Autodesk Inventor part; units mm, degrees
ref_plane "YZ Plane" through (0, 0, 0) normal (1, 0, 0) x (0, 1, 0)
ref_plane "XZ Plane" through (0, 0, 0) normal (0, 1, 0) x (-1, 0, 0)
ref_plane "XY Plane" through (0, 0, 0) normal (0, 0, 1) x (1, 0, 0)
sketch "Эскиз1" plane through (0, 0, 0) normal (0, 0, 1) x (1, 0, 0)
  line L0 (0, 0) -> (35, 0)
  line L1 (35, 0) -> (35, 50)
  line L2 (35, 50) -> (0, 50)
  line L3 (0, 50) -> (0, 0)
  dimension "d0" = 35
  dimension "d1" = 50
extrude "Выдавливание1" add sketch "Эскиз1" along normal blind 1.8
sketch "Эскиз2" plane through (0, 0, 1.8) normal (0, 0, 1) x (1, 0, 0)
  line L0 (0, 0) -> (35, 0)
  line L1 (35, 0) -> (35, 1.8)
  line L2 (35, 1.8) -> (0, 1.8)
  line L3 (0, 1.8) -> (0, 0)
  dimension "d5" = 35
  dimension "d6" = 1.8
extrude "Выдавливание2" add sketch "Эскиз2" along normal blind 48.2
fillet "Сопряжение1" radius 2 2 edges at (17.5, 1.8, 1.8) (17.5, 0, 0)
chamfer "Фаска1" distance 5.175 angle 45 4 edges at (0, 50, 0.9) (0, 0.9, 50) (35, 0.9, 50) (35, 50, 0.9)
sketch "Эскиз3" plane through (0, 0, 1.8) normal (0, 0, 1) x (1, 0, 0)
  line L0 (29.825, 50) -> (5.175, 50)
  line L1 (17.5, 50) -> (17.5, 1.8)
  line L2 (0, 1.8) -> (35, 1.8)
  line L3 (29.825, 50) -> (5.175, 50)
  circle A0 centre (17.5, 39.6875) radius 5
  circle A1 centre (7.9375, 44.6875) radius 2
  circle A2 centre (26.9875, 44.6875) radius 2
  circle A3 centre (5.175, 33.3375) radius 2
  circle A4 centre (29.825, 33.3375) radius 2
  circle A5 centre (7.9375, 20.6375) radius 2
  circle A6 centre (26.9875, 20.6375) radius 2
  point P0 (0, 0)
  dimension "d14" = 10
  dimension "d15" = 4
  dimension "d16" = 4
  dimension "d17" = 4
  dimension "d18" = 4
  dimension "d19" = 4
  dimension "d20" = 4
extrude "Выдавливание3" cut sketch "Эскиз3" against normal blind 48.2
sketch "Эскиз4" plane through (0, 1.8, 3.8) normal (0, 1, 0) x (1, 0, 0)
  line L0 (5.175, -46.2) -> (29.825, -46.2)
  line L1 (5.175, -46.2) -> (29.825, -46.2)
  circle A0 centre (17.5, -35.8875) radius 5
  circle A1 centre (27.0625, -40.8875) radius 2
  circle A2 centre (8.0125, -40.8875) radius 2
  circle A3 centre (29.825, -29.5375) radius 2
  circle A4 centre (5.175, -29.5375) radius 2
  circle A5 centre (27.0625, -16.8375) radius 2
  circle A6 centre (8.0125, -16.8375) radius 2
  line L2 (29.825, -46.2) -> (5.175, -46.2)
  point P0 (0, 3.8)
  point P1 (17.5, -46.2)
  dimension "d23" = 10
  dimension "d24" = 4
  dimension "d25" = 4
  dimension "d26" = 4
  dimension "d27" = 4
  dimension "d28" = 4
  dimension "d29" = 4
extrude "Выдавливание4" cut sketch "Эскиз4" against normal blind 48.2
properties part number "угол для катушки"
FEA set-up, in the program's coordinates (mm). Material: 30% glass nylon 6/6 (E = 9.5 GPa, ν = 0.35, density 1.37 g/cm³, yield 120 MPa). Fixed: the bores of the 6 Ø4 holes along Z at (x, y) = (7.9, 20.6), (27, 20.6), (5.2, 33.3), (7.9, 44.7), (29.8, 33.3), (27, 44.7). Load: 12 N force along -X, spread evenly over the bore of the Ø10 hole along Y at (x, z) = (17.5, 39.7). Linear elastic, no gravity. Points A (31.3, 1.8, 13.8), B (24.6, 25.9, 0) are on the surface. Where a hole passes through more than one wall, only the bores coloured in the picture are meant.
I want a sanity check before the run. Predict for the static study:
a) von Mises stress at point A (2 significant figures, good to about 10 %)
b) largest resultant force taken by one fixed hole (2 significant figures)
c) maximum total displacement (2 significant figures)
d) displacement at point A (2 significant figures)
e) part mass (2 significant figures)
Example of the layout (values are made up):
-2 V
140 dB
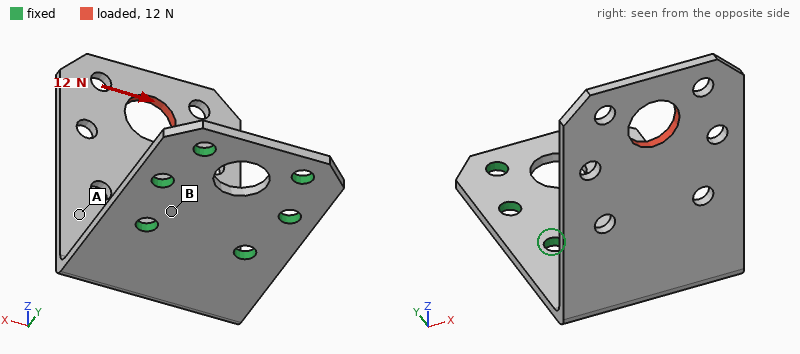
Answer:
3.9 MPa
24 N
0.78 mm
0.30 mm
7.6 g
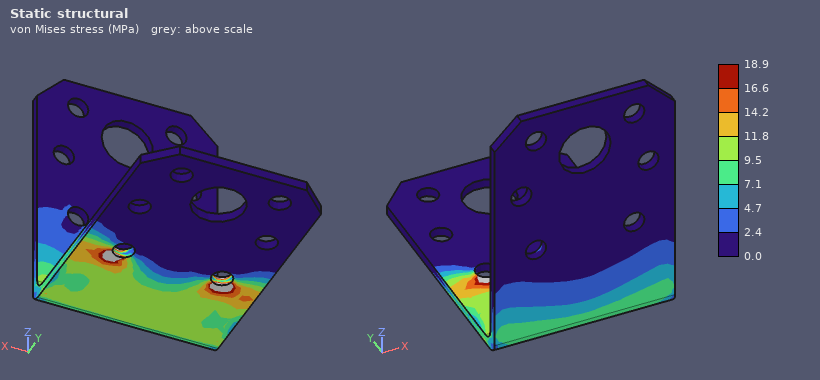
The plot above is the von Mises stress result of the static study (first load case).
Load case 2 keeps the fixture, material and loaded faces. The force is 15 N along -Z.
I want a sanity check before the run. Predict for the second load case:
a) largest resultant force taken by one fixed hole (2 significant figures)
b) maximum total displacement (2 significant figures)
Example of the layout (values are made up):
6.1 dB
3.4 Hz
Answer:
9.4 N
0.78 mm
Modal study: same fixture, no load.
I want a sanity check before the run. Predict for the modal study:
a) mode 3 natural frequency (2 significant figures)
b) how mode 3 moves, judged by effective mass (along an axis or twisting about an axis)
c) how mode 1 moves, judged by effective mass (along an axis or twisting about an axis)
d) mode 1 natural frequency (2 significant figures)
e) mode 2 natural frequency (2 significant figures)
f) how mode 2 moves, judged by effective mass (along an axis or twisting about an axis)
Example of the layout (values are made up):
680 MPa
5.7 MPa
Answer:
910 Hz
along Z
along Y
230 Hz
490 Hz
along X
